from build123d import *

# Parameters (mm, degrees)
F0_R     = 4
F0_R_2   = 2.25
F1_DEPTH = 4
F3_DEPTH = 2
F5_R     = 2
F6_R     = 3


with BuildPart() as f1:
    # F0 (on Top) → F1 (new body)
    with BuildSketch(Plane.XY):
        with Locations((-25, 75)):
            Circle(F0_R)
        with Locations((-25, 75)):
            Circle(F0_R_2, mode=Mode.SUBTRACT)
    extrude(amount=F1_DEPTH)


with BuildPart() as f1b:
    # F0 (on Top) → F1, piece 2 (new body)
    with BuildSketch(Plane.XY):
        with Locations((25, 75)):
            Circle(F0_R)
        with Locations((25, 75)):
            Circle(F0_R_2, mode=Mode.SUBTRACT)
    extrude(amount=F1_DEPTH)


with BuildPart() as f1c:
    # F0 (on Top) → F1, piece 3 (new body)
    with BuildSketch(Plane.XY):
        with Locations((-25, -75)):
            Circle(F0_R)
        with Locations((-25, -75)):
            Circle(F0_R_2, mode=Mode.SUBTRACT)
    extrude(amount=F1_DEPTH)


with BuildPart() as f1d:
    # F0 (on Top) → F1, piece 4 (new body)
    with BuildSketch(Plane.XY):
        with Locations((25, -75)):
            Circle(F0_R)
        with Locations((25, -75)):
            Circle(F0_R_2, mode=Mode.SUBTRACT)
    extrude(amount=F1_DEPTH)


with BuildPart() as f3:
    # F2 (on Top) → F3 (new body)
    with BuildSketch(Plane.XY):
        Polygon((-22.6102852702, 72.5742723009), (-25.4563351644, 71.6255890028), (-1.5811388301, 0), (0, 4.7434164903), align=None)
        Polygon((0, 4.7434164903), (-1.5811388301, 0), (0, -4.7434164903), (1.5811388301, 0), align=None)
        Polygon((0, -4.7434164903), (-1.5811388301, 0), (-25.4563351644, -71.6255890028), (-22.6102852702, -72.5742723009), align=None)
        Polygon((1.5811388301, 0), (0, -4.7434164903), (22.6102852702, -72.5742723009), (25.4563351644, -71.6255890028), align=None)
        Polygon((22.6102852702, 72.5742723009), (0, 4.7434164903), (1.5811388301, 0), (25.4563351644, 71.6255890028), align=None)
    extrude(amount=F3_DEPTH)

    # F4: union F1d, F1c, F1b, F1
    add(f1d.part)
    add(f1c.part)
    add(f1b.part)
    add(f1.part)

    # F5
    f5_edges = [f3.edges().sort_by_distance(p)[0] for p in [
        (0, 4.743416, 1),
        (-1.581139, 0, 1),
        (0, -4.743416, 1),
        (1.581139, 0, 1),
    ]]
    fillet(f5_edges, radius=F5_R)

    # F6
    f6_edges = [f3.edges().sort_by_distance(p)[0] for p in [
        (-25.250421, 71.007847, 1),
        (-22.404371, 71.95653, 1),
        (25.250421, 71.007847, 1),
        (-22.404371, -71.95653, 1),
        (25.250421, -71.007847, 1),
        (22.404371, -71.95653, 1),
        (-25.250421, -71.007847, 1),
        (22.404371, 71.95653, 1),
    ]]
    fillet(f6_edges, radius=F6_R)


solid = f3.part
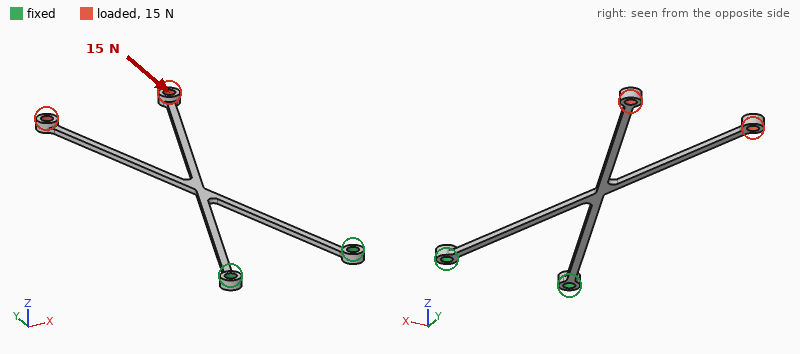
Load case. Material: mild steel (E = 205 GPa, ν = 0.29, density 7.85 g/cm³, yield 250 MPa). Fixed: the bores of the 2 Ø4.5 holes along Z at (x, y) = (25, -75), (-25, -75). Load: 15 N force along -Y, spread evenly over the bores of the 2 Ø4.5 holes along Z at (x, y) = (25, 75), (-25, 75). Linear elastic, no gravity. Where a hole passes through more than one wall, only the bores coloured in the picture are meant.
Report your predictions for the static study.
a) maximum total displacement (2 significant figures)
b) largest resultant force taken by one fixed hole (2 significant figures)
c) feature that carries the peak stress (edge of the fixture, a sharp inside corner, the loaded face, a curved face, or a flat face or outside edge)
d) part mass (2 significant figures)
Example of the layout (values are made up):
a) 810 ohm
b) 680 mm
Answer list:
a) 0.40 mm
b) 7.9 N
c) a curved face
d) 19 g
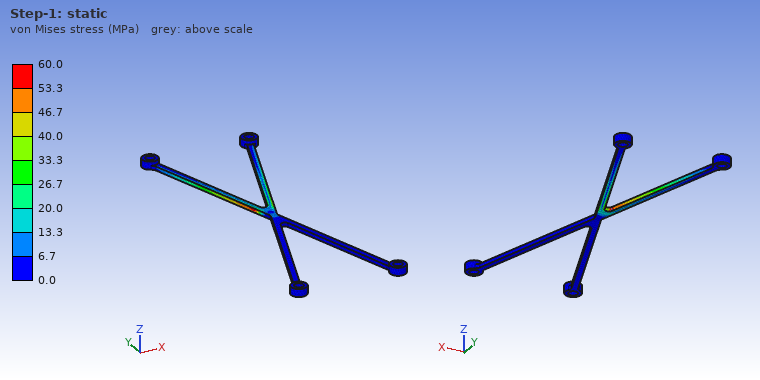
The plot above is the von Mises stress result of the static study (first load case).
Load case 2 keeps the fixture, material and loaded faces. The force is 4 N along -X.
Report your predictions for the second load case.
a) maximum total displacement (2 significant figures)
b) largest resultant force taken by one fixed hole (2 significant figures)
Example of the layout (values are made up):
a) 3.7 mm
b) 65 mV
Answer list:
a) 0.54 mm
b) 15 N
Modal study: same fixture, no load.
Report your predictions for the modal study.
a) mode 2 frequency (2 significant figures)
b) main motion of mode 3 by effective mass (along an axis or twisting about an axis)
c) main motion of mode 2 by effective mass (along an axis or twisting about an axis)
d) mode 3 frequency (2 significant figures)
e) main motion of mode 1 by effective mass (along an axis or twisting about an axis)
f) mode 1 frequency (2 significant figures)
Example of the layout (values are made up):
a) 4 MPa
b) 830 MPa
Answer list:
a) 180 Hz
b) along X
c) twisting about Y
d) 220 Hz
e) along Z
f) 59 Hz
